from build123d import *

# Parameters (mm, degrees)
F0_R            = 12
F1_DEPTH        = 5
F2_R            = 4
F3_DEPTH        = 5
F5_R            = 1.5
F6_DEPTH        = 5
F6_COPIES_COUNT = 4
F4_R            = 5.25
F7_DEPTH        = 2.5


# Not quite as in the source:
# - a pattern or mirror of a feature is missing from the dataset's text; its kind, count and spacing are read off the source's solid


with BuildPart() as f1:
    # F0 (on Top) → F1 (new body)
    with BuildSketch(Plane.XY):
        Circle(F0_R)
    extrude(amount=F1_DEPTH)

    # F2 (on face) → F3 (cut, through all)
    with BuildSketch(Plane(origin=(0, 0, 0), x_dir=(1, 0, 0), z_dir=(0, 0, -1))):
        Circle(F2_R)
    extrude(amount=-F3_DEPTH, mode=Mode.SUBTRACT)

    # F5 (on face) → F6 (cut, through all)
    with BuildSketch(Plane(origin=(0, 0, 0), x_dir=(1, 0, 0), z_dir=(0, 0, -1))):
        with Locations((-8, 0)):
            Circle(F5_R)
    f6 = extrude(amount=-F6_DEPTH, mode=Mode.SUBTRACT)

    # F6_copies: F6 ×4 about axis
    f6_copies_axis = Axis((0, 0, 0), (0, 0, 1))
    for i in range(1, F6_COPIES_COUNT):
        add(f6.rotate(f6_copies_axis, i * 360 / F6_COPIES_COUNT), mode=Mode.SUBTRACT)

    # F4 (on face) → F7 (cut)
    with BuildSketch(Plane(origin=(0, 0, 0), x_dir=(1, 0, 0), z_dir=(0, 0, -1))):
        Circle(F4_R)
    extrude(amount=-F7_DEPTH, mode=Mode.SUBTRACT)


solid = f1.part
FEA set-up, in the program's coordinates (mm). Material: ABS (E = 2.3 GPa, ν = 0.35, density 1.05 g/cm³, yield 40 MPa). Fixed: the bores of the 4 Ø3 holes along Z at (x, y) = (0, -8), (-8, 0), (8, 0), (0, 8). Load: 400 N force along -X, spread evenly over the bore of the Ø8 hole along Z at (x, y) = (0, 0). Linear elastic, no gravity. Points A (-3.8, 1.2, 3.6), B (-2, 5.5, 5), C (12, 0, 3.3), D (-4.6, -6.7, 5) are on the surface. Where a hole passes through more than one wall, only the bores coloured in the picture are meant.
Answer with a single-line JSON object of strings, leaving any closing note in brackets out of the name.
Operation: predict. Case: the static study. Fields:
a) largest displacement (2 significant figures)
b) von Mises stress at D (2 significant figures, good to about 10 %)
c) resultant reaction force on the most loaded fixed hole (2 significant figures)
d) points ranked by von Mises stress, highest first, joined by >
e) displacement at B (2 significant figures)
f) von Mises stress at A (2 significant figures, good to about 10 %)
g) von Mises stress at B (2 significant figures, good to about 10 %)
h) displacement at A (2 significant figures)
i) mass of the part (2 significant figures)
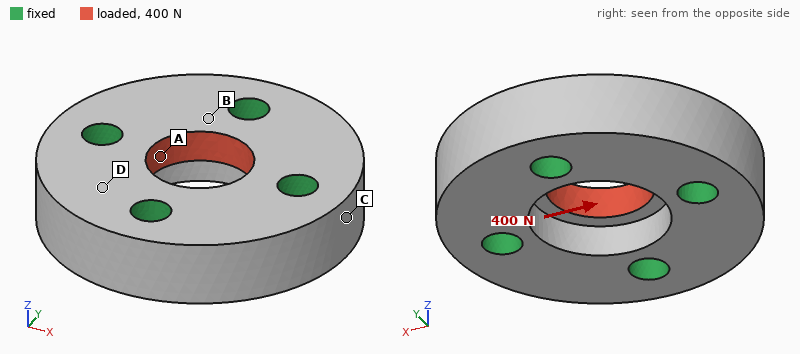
{"largest displacement": "16 µm", "von Mises stress at D": "2.2 MPa", "resultant reaction force on the most loaded fixed hole": "120 N", "points ranked by von Mises stress, highest first, joined by >": "A > B > D > C", "displacement at B": "6.7 µm", "von Mises stress at A": "6.6 MPa", "von Mises stress at B": "3.3 MPa", "displacement at A": "10 µm", "mass of the part": "1.9 g"}
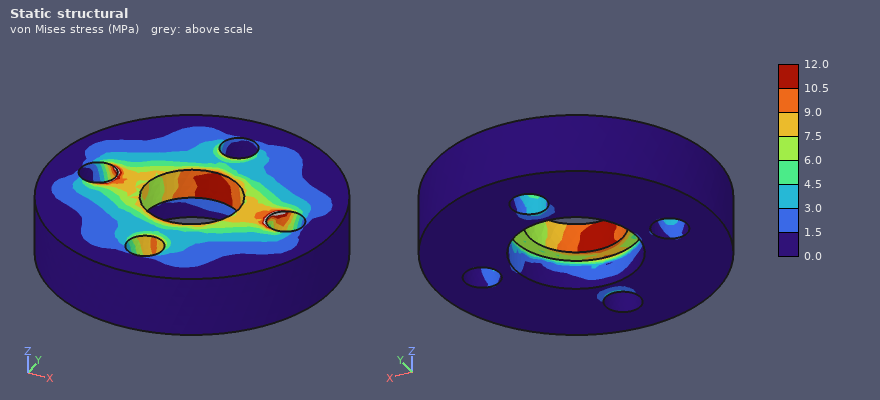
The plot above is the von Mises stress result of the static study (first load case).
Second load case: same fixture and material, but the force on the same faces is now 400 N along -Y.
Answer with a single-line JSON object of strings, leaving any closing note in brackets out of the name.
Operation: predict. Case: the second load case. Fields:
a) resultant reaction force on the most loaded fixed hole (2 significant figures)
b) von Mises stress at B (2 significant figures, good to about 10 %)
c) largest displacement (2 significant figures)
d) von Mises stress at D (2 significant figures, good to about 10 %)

{"resultant reaction force on the most loaded fixed hole": "120 N", "von Mises stress at B": "6.3 MPa", "largest displacement": "16 µm", "von Mises stress at D": "2.4 MPa"}
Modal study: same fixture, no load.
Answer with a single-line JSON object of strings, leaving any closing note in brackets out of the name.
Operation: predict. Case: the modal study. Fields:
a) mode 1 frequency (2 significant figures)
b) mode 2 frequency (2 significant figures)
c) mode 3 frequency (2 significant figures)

{"mode 1 frequency": "24 kHz", "mode 2 frequency": "24 kHz", "mode 3 frequency": "24 kHz"}
